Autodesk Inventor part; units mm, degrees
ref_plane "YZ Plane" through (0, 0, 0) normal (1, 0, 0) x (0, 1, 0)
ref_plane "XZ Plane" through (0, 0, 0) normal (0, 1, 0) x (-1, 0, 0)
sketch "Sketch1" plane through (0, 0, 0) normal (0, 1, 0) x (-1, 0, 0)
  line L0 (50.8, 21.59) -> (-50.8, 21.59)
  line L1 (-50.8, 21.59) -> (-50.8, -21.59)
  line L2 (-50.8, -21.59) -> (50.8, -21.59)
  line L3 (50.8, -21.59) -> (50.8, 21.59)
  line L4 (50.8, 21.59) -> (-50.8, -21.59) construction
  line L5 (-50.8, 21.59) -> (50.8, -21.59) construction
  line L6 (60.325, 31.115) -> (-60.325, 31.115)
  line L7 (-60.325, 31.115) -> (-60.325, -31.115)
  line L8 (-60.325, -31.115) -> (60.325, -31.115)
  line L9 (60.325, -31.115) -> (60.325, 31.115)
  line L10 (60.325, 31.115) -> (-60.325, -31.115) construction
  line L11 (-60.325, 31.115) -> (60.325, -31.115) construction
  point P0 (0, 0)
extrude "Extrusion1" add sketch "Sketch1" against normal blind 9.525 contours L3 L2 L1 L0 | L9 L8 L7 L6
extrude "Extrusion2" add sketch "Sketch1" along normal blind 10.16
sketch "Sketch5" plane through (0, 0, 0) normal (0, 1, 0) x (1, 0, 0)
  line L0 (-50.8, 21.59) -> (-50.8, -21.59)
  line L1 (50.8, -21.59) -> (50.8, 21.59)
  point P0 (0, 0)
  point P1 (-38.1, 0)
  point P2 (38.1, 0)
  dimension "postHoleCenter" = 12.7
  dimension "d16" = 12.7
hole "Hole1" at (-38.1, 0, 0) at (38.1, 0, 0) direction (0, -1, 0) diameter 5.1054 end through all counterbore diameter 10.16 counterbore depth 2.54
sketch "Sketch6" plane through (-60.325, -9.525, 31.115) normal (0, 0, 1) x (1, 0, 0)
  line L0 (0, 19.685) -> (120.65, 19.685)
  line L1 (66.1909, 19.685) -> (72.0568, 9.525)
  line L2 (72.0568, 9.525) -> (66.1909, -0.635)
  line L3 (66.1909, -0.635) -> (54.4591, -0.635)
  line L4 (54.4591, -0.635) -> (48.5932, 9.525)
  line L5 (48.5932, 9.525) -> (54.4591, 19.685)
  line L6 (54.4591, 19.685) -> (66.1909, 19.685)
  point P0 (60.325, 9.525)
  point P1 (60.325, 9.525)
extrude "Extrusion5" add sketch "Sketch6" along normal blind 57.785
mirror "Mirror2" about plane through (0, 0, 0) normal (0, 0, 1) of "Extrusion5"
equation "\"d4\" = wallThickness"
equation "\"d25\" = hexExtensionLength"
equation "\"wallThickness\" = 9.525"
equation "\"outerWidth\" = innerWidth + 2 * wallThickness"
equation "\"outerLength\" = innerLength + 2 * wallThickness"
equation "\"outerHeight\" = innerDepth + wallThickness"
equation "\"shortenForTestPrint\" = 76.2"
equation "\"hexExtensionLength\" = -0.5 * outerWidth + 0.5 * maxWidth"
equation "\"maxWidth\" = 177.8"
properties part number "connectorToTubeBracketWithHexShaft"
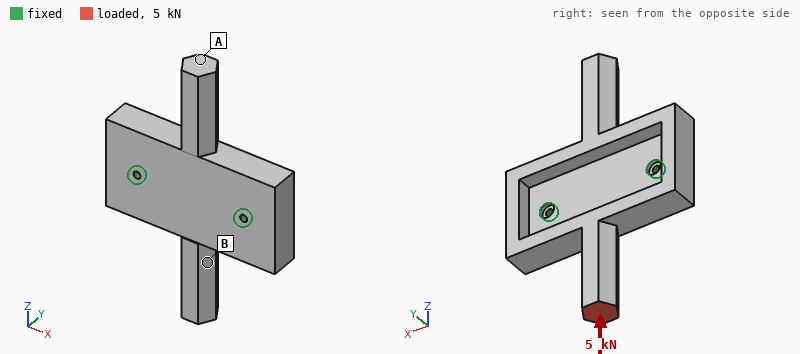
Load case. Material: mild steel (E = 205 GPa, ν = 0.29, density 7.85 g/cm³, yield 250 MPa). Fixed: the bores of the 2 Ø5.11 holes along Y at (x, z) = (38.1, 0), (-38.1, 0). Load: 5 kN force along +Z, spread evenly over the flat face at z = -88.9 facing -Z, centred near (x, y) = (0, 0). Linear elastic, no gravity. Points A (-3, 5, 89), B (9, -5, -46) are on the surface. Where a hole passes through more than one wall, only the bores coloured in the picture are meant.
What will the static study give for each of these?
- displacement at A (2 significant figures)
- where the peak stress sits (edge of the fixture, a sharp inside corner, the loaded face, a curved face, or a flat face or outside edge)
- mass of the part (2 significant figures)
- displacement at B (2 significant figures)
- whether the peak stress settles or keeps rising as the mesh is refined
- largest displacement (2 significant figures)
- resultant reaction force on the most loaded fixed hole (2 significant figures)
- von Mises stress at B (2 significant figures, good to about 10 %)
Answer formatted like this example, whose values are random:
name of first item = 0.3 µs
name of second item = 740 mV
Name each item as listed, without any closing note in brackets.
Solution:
displacement at A = 32 µm
where the peak stress sits = edge of the fixture
mass of the part = 1.1 kg
displacement at B = 30 µm
whether the peak stress settles or keeps rising as the mesh is refined = keeps rising
largest displacement = 67 µm
resultant reaction force on the most loaded fixed hole = 2.5 kN
von Mises stress at B = 14 MPa
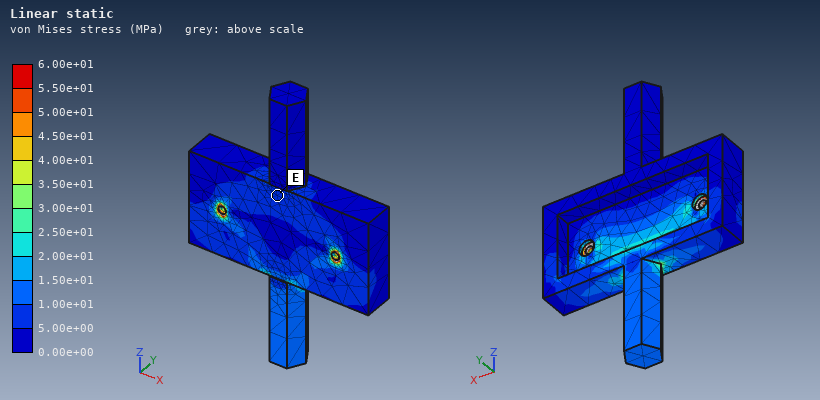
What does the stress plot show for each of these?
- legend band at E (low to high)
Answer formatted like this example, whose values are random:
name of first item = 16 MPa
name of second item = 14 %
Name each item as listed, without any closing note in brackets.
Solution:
legend band at E = 5.00e+00 to 1.00e+01 MPa
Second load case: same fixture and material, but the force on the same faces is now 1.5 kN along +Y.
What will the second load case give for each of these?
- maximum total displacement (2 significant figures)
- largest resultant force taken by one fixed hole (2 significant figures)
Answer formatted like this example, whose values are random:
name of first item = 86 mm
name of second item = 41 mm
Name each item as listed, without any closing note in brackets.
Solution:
maximum total displacement = 0.37 mm
largest resultant force taken by one fixed hole = 810 N
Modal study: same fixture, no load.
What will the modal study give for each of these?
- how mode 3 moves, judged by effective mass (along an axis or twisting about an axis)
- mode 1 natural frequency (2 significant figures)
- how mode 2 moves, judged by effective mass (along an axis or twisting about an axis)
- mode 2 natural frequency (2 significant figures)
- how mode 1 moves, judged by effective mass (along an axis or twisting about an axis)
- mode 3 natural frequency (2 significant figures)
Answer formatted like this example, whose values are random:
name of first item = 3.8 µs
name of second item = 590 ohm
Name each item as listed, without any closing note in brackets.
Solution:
how mode 3 moves, judged by effective mass = twisting about Y
mode 1 natural frequency = 960 Hz
how mode 2 moves, judged by effective mass = along Y
mode 2 natural frequency = 1600 Hz
how mode 1 moves, judged by effective mass = twisting about X
mode 3 natural frequency = 3200 Hz
